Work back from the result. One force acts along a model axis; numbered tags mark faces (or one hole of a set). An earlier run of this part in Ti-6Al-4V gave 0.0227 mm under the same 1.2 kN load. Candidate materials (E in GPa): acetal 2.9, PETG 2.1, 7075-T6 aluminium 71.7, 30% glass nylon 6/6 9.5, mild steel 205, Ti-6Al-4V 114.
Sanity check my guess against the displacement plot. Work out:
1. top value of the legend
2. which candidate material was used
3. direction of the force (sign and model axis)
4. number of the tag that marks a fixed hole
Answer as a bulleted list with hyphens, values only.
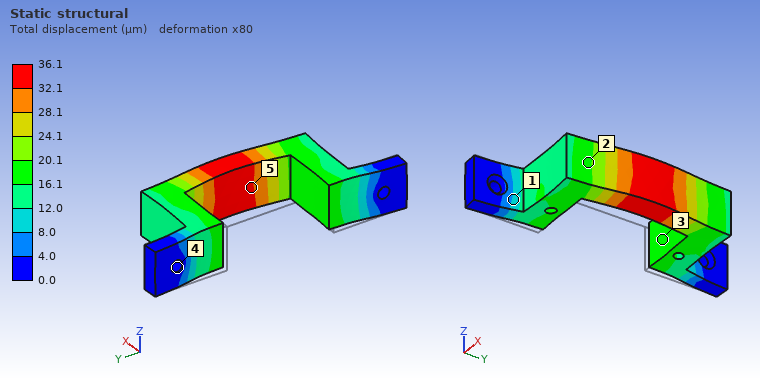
- 36.1 µm
- 7075-T6 aluminium
- +X
- 4
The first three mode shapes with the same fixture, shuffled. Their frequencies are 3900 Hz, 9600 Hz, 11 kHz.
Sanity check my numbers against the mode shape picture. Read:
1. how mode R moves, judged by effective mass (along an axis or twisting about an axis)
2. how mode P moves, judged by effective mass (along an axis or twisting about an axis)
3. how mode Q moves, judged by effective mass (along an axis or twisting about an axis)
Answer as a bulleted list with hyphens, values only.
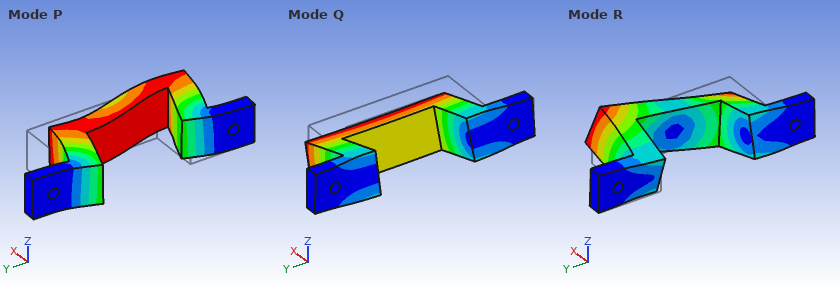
- twisting about X
- along Y
- along Z
